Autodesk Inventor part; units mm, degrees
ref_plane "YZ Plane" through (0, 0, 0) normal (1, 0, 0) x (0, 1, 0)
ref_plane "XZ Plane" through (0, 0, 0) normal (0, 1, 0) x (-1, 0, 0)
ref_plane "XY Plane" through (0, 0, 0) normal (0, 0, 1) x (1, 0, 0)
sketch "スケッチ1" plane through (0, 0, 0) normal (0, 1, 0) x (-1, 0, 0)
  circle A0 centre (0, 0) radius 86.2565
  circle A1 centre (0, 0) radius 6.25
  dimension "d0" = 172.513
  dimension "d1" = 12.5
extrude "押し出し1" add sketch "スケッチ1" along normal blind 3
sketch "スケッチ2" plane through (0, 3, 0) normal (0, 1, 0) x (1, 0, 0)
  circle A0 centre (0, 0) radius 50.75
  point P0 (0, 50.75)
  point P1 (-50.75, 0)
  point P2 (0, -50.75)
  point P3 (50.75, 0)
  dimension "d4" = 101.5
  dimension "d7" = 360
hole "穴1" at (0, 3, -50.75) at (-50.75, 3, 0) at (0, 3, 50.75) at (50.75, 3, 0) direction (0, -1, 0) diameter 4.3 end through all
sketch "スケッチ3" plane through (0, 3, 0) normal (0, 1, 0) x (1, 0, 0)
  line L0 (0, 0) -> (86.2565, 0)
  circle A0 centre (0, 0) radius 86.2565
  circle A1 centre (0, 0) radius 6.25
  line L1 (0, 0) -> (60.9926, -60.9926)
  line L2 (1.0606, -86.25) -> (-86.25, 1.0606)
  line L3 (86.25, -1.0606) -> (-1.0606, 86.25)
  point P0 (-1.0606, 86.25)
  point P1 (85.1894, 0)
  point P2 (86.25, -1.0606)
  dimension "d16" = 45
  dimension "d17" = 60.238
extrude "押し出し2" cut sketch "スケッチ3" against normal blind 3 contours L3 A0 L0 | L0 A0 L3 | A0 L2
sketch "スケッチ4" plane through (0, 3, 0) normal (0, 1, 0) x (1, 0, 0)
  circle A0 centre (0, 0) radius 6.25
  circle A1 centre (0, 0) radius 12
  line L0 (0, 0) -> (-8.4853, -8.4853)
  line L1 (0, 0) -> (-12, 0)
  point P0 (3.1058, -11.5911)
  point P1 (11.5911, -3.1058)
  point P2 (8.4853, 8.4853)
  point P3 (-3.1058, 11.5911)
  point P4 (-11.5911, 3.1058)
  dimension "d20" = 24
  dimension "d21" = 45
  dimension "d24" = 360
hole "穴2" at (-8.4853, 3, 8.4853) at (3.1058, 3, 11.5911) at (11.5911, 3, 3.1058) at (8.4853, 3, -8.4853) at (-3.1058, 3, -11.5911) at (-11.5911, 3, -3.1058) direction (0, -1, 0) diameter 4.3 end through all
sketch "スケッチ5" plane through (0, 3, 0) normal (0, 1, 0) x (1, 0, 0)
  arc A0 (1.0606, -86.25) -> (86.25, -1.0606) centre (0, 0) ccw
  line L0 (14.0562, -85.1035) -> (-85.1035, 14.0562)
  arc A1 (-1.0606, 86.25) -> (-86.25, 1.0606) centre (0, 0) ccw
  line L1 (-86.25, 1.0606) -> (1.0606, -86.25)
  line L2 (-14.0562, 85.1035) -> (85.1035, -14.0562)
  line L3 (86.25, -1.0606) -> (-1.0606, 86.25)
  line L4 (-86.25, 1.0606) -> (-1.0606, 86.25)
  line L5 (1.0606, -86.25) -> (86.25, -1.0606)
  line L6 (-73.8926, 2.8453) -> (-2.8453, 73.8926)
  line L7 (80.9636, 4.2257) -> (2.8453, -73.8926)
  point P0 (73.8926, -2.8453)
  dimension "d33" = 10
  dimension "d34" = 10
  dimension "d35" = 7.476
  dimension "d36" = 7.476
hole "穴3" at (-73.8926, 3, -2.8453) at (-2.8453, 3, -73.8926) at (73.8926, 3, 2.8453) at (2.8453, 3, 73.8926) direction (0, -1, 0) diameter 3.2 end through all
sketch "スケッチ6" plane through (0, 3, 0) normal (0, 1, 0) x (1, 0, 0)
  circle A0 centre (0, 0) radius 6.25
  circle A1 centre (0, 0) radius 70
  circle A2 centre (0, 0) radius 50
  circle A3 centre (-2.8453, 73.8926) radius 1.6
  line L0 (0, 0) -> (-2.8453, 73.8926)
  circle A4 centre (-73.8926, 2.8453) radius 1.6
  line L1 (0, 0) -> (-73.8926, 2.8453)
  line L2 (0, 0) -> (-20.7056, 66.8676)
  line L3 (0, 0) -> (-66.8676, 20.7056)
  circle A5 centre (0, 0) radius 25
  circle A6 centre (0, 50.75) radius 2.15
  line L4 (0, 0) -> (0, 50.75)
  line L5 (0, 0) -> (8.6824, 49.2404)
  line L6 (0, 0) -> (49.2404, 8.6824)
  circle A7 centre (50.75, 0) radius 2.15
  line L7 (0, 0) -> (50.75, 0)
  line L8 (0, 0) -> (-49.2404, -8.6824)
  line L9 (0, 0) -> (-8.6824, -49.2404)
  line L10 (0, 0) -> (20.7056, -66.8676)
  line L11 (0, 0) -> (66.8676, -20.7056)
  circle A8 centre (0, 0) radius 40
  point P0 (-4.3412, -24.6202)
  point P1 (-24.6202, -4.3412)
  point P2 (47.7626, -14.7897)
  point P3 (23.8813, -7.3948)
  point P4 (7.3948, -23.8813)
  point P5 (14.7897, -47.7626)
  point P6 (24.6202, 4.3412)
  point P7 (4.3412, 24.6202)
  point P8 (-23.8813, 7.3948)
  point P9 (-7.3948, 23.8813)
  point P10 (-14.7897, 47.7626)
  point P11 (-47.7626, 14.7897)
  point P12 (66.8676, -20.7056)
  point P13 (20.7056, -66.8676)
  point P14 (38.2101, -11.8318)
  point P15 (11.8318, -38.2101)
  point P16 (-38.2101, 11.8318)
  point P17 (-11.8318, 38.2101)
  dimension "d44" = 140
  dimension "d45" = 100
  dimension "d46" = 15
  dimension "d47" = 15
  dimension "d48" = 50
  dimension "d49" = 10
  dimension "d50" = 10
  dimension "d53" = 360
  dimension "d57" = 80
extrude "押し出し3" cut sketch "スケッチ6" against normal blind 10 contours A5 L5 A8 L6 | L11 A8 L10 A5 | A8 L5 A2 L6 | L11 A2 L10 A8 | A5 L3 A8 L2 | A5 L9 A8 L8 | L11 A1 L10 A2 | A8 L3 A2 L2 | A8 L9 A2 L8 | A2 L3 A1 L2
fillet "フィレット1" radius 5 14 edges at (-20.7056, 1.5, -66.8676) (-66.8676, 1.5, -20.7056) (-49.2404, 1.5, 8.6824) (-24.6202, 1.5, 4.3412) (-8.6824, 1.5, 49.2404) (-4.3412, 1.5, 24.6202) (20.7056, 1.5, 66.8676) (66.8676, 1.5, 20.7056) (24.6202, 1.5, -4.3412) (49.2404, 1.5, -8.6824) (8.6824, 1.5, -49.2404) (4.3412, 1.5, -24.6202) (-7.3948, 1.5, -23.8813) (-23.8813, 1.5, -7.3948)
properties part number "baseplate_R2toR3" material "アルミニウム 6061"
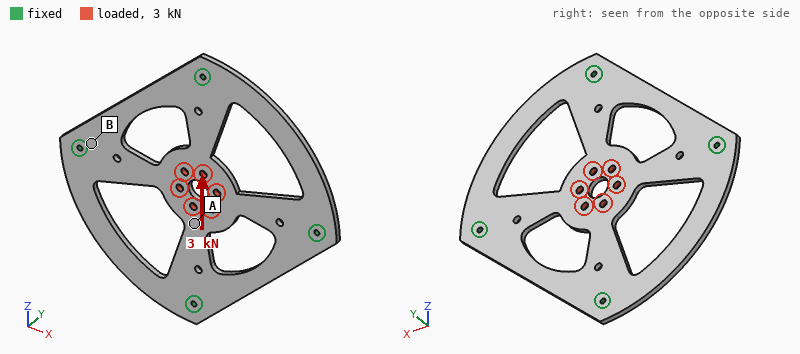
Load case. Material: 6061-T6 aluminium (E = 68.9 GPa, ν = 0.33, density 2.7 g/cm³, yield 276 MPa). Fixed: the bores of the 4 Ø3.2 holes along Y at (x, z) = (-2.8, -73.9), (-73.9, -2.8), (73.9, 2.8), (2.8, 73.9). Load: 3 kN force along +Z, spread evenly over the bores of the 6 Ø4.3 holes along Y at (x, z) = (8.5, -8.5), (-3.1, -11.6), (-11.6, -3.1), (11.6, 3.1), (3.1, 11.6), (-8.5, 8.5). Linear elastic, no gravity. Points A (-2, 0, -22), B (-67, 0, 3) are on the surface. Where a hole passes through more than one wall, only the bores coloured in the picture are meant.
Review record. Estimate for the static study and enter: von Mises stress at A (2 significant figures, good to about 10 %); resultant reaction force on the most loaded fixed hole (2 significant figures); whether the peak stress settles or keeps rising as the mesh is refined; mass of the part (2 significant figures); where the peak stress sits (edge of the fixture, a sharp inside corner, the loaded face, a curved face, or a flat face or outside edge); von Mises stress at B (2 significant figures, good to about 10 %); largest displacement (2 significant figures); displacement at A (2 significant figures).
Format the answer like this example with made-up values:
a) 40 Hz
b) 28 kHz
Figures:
a) 25 MPa
b) 1.2 kN
c) keeps rising
d) 99 g
e) edge of the fixture
f) 5.1 MPa
g) 27 µm
h) 19 µm
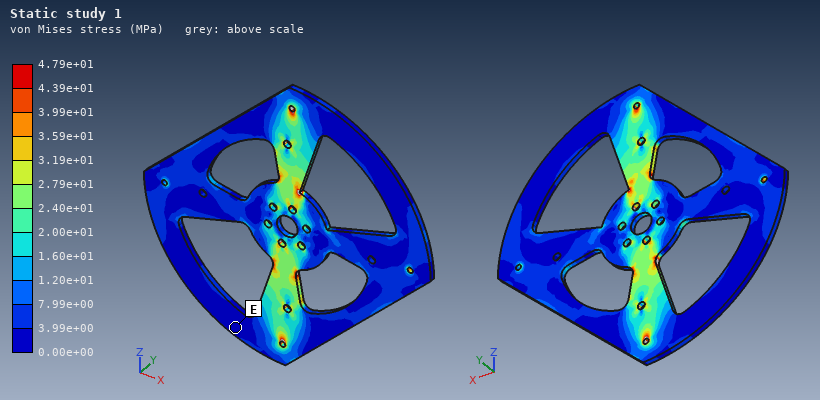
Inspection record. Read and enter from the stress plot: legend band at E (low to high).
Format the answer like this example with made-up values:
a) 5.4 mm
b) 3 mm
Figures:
a) 0.00e+00 to 3.99e+00 MPa
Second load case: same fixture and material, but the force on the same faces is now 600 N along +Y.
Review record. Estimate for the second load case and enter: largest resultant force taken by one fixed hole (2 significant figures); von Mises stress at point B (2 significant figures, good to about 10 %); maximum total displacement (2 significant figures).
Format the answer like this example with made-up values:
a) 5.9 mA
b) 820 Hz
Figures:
a) 150 N
b) 76 MPa
c) 1.1 mm
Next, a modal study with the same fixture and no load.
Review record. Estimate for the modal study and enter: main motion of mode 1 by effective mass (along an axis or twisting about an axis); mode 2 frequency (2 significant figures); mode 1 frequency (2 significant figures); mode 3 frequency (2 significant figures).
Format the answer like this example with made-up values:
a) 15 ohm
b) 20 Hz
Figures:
a) along Y
b) 1200 Hz
c) 900 Hz
d) 1200 Hz
